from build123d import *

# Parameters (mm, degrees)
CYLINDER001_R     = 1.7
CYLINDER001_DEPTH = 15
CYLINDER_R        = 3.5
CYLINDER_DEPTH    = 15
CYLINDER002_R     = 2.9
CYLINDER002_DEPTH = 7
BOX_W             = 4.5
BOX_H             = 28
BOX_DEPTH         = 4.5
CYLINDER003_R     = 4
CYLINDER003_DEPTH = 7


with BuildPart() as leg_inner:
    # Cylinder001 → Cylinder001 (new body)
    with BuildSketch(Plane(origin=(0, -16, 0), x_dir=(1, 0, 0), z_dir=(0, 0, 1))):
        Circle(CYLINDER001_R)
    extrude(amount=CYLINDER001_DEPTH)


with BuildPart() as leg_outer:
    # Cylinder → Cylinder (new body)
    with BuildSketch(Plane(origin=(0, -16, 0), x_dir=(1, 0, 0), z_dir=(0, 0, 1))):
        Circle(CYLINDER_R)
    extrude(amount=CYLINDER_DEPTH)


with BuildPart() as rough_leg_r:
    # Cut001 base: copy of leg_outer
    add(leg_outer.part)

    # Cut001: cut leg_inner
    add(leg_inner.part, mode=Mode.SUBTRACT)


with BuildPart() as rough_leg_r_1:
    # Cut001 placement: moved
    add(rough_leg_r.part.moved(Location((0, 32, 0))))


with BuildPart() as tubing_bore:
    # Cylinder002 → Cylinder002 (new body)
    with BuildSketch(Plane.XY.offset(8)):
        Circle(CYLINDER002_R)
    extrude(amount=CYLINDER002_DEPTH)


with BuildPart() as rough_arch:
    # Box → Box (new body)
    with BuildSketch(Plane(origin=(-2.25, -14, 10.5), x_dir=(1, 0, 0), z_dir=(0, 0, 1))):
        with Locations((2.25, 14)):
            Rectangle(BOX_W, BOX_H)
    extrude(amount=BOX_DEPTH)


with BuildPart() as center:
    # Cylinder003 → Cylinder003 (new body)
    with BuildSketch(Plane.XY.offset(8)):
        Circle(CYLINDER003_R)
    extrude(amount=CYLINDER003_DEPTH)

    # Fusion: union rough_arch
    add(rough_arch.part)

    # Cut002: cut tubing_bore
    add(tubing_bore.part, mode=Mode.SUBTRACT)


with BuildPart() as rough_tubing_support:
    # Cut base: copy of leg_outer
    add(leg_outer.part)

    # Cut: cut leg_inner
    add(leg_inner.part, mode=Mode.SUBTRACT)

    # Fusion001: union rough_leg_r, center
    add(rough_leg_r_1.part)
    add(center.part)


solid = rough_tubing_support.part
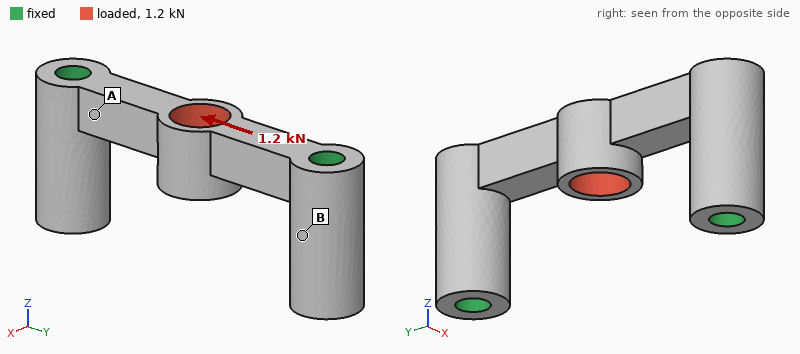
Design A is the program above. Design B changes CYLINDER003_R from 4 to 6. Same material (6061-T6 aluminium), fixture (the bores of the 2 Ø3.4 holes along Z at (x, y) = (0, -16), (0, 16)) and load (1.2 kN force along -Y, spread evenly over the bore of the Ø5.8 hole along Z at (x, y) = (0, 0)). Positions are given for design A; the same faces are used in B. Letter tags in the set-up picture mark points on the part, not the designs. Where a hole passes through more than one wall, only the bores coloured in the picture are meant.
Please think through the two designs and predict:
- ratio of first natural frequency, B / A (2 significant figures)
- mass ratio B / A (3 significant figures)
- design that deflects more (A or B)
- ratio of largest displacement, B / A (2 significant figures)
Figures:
0.74
1.25
A
0.54
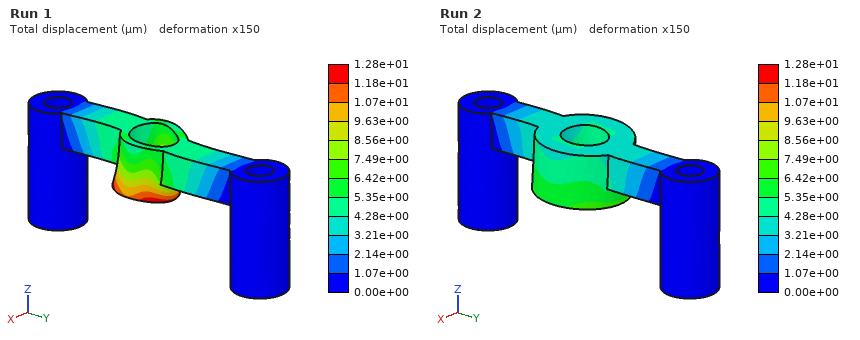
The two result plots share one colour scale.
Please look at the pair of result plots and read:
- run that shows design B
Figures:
Run 2
